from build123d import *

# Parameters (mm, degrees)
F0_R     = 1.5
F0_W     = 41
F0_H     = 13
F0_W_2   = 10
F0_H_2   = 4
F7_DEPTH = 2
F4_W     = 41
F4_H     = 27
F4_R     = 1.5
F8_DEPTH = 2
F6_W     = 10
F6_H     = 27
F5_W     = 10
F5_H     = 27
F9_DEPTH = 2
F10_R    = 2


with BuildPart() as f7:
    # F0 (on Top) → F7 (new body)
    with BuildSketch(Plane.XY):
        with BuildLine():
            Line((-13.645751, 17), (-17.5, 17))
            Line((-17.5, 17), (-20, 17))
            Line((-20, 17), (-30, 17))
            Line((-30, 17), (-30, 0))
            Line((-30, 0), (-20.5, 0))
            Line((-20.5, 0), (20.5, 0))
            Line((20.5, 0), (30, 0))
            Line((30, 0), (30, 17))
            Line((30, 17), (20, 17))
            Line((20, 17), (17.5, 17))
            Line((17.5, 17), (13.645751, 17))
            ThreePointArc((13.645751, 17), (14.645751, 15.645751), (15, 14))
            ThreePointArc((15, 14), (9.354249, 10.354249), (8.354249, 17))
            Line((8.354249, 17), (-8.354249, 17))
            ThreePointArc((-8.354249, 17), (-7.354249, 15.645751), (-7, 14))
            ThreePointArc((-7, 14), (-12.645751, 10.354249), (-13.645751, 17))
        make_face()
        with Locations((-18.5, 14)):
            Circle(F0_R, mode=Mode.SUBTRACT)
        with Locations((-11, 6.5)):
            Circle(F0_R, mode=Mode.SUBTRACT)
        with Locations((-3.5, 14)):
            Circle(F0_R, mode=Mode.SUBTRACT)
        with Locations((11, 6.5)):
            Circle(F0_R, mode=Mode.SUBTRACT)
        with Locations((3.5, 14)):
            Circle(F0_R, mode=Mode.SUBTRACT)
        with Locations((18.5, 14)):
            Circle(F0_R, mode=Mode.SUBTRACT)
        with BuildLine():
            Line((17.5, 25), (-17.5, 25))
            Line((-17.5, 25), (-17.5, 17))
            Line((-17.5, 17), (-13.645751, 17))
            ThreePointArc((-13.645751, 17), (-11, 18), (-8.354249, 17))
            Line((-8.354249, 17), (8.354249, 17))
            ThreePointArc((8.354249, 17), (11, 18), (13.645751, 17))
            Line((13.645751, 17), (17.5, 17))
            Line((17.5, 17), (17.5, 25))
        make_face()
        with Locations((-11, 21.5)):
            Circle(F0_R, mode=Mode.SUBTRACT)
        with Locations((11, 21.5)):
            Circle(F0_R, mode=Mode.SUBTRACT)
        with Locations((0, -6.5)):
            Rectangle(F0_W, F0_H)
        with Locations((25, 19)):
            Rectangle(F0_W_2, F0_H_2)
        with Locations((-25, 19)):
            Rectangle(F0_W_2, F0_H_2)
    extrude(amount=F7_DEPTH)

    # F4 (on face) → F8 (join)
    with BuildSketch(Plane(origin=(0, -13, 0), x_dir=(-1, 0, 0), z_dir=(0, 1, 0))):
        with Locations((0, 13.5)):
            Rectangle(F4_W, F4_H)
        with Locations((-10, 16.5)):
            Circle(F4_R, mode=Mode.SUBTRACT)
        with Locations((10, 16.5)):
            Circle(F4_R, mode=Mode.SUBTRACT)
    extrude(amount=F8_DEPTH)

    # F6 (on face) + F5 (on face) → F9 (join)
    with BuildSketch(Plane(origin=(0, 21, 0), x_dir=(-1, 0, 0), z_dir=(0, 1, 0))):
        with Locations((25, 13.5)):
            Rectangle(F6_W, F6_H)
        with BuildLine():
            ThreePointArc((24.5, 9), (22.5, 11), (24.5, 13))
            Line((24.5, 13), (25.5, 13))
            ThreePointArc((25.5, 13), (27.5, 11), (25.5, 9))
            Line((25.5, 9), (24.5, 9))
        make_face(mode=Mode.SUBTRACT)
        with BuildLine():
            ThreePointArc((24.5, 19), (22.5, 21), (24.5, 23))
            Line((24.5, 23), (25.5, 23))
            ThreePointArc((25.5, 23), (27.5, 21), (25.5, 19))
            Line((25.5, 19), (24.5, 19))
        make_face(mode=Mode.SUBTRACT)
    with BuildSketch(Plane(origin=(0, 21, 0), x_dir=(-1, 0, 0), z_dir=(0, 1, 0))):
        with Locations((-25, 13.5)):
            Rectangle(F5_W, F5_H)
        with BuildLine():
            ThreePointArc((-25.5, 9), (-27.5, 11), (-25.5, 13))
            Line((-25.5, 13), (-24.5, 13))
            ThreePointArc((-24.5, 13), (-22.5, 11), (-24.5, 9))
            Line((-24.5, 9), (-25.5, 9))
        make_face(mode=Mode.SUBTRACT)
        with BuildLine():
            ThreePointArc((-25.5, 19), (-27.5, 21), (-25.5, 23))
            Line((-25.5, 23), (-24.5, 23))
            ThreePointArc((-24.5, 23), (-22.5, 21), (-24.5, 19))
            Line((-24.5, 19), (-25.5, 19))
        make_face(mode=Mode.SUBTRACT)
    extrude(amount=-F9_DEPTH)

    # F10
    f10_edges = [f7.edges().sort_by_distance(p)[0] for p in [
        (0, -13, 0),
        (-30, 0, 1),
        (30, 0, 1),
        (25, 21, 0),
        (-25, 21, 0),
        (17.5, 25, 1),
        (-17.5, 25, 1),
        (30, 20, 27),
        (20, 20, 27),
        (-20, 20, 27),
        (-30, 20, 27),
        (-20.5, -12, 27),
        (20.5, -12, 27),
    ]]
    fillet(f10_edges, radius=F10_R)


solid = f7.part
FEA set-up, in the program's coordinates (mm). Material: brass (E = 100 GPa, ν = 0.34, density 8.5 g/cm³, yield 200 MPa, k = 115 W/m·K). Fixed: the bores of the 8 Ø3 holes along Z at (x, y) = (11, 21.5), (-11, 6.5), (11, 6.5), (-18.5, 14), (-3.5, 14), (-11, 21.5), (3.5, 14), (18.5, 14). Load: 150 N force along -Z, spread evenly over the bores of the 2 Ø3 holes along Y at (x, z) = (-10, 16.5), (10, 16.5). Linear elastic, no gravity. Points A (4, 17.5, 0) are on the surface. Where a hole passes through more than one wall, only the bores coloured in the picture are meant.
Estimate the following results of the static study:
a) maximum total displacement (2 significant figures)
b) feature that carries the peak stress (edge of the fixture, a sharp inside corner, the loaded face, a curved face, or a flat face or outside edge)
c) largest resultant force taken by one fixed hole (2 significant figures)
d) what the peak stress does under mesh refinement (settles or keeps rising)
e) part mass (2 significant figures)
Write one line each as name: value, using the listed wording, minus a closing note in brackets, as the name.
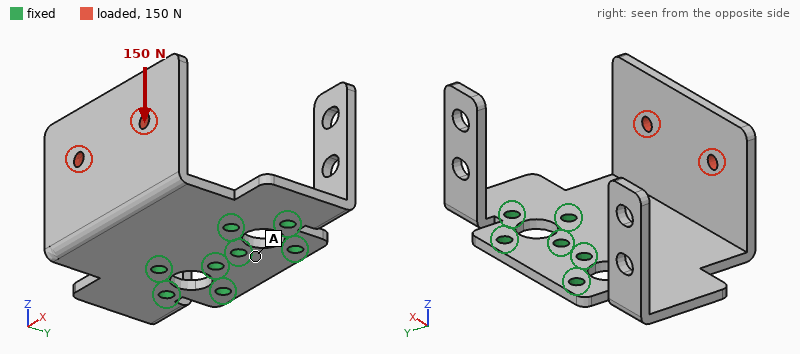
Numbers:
maximum total displacement: 0.24 mm
feature that carries the peak stress: edge of the fixture
largest resultant force taken by one fixed hole: 140 N
what the peak stress does under mesh refinement: keeps rising
part mass: 54 g
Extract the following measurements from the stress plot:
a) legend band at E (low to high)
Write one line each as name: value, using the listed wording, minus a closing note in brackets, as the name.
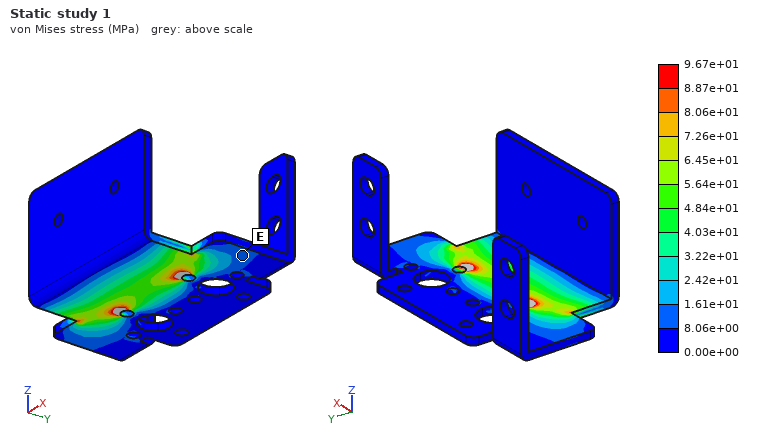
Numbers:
legend band at E: 8.06e+00 to 1.61e+01 MPa
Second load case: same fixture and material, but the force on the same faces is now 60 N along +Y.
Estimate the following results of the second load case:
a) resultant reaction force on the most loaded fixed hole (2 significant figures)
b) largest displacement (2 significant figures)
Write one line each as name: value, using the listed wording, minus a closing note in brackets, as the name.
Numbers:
resultant reaction force on the most loaded fixed hole: 34 N
largest displacement: 0.20 mm
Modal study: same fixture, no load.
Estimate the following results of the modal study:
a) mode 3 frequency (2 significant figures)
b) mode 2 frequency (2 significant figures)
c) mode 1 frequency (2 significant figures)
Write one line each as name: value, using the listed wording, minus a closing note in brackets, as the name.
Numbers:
mode 3 frequency: 1200 Hz
mode 2 frequency: 1200 Hz
mode 1 frequency: 790 Hz
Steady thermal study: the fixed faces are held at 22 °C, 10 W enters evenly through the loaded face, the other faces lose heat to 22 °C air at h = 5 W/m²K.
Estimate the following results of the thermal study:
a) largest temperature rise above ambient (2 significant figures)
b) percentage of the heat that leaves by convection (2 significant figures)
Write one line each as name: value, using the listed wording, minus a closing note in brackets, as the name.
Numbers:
largest temperature rise above ambient: 39 K
percentage of the heat that leaves by convection: 4.4 %
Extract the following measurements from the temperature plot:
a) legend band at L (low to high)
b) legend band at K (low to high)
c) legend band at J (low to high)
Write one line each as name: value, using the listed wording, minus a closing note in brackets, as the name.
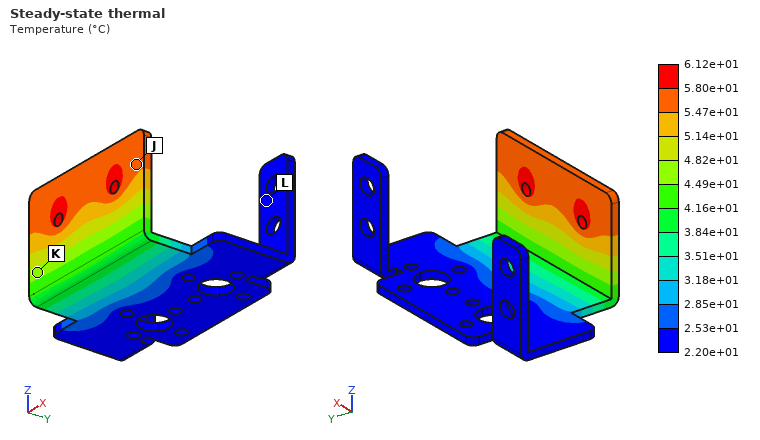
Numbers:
legend band at L: 2.20e+01 to 2.53e+01 °C
legend band at K: 4.49e+01 to 4.82e+01 °C
legend band at J: 5.47e+01 to 5.80e+01 °C
